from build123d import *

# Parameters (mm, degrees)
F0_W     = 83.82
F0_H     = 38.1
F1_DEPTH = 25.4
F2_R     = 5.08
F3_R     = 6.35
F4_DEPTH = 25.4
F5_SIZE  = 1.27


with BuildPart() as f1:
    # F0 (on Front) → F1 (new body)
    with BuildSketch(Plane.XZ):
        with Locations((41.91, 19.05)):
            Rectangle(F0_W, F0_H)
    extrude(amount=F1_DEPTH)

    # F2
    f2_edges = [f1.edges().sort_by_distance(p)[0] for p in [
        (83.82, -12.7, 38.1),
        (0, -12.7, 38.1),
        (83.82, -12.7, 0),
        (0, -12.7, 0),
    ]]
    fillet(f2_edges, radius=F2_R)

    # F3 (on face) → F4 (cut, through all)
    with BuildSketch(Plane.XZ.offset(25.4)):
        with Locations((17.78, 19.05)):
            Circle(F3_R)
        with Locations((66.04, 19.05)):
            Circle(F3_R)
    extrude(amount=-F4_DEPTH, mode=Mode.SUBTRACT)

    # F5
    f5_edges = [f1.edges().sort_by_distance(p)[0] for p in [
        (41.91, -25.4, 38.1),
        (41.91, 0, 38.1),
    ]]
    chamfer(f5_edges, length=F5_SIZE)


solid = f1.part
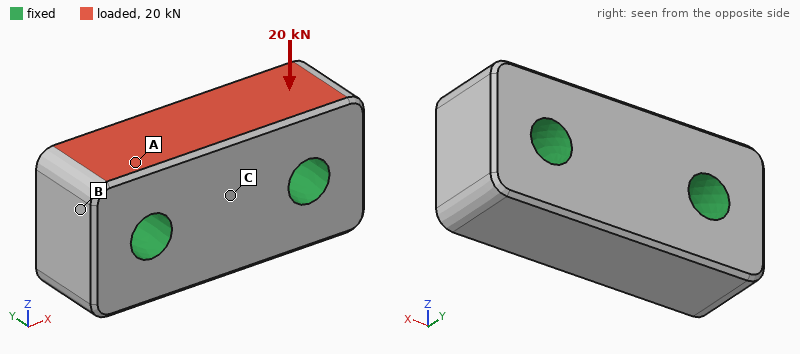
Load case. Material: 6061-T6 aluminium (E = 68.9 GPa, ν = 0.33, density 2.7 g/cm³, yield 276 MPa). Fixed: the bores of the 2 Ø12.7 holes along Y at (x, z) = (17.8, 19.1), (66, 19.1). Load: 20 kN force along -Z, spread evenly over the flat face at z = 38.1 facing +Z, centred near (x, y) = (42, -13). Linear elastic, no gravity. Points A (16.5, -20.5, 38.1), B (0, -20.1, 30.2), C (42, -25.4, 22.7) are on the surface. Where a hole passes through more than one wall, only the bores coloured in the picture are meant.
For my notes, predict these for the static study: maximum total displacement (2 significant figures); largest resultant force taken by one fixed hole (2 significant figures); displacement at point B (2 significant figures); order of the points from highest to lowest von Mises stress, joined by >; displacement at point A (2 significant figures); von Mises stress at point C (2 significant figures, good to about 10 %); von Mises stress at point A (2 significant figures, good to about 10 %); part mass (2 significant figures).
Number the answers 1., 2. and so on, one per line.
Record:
1. 5.1 µm
2. 10 kN
3. 1.5 µm
4. A > C > B
5. 2.4 µm
6. 5.1 MPa
7. 13 MPa
8. 200 g
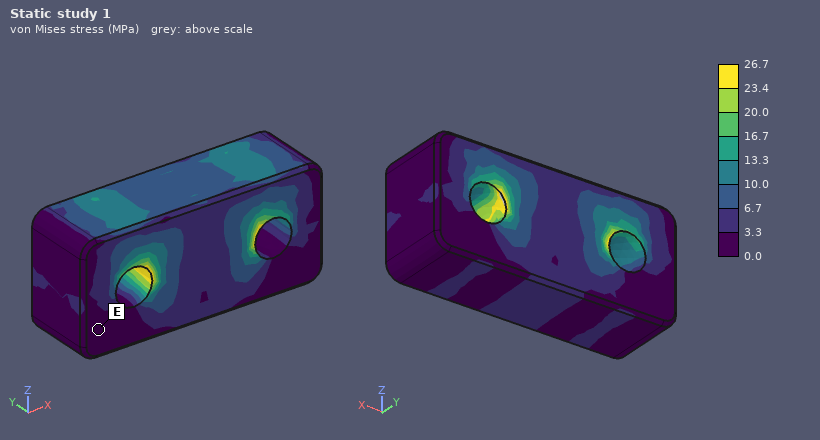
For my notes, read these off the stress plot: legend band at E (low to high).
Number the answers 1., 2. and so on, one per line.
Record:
1. 0.0 to 3.3 MPa
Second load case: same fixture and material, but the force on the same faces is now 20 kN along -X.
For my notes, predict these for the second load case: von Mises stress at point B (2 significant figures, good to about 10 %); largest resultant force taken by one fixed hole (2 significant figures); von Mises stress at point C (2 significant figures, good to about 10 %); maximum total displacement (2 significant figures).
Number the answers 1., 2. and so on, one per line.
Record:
1. 9.6 MPa
2. 11 kN
3. 12 MPa
4. 10 µm
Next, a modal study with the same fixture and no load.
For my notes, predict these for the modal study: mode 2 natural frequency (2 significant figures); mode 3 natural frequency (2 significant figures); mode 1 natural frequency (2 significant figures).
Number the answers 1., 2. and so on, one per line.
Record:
1. 28 kHz
2. 28 kHz
3. 28 kHz
